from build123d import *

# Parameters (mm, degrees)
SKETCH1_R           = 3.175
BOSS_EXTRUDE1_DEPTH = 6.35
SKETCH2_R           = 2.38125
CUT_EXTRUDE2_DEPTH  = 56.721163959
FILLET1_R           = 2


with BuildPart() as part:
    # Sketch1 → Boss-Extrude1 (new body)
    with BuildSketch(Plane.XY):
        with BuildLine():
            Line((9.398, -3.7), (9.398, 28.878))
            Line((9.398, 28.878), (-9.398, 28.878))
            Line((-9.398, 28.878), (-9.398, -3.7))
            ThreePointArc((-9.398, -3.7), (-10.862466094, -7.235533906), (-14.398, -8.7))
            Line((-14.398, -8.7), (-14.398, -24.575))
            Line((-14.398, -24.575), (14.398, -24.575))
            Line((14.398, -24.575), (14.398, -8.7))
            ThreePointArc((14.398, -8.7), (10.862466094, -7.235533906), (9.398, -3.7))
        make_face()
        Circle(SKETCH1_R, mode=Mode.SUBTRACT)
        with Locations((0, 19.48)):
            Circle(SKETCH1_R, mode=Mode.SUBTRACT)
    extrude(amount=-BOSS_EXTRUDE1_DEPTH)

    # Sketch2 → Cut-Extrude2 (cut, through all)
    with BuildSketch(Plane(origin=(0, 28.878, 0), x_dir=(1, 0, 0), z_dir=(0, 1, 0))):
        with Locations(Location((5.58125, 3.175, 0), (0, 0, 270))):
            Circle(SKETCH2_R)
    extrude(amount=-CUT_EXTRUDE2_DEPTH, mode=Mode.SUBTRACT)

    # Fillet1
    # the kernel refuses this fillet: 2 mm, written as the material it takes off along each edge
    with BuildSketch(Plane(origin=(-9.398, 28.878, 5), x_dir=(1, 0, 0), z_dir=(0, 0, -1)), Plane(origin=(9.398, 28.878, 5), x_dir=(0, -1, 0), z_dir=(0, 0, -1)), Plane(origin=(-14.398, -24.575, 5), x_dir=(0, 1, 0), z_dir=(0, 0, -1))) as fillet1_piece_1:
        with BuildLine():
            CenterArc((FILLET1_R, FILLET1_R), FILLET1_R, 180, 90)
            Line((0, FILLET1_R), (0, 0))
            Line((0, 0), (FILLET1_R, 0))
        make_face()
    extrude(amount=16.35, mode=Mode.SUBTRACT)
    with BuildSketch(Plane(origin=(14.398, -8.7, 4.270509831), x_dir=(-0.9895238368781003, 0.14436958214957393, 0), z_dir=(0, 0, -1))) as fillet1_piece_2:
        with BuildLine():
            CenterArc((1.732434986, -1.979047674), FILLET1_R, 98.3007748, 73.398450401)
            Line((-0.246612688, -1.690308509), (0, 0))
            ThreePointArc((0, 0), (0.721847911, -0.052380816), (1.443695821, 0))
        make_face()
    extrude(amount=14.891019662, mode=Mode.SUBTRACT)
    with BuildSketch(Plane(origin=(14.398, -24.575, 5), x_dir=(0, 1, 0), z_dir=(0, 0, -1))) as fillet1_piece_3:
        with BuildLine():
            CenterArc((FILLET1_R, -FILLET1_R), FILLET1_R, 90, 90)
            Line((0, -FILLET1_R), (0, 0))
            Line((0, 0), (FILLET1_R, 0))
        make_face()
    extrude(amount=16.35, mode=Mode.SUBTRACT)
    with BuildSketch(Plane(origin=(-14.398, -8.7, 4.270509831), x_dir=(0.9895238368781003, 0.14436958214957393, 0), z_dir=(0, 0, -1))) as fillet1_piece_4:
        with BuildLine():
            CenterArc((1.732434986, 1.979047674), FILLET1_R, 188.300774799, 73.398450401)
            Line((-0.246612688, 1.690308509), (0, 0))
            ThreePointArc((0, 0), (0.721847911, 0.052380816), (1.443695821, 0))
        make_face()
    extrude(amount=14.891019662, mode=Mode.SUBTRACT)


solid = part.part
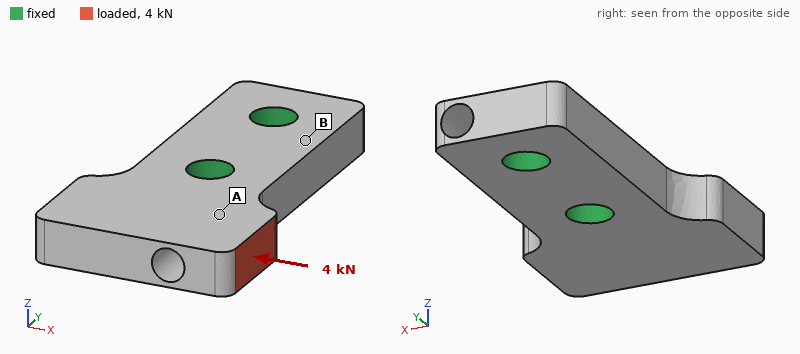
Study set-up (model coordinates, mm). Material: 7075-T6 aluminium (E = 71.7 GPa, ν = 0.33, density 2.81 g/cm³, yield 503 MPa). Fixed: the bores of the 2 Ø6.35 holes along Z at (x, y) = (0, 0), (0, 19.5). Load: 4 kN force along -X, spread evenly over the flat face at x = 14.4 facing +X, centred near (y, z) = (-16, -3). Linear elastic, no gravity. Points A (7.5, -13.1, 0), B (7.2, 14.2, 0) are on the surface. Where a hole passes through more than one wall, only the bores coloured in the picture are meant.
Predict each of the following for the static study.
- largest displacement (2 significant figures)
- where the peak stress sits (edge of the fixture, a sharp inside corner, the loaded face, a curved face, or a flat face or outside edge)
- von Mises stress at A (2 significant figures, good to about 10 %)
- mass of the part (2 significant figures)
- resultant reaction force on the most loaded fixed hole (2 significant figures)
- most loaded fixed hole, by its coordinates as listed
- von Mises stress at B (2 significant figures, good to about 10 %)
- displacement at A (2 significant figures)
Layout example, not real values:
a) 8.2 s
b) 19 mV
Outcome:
a) 0.13 mm
b) edge of the fixture
c) 160 MPa
d) 17 g
e) 5.3 kN
f) (0, 0)
g) 44 MPa
h) 0.070 mm
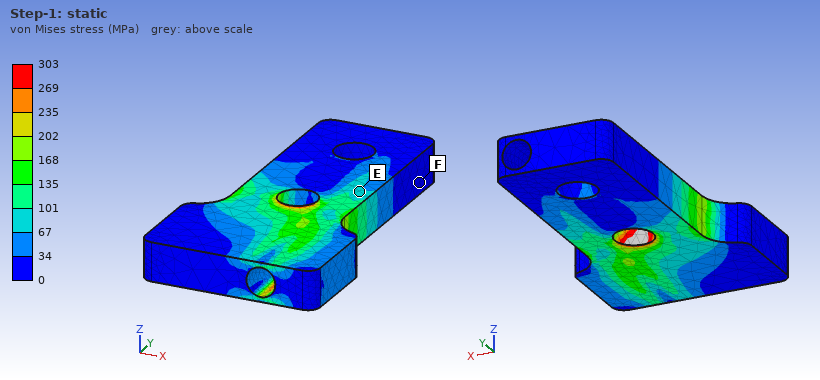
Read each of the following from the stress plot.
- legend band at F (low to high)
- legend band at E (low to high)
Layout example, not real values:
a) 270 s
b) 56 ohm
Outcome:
a) 0 to 34 MPa
b) 67 to 101 MPa
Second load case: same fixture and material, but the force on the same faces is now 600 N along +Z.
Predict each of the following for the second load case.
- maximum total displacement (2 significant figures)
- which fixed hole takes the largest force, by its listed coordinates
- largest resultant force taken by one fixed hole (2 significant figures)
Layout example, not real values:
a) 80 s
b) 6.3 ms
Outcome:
a) 0.11 mm
b) (0, 0)
c) 650 N
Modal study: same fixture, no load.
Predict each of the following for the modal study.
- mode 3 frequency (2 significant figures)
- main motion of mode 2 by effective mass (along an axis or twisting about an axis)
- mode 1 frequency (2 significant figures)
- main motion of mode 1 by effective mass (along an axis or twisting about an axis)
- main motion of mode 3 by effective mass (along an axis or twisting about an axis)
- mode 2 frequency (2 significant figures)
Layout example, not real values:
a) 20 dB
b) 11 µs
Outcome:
a) 12 kHz
b) twisting about Y
c) 7700 Hz
d) along Z
e) along X
f) 11 kHz
